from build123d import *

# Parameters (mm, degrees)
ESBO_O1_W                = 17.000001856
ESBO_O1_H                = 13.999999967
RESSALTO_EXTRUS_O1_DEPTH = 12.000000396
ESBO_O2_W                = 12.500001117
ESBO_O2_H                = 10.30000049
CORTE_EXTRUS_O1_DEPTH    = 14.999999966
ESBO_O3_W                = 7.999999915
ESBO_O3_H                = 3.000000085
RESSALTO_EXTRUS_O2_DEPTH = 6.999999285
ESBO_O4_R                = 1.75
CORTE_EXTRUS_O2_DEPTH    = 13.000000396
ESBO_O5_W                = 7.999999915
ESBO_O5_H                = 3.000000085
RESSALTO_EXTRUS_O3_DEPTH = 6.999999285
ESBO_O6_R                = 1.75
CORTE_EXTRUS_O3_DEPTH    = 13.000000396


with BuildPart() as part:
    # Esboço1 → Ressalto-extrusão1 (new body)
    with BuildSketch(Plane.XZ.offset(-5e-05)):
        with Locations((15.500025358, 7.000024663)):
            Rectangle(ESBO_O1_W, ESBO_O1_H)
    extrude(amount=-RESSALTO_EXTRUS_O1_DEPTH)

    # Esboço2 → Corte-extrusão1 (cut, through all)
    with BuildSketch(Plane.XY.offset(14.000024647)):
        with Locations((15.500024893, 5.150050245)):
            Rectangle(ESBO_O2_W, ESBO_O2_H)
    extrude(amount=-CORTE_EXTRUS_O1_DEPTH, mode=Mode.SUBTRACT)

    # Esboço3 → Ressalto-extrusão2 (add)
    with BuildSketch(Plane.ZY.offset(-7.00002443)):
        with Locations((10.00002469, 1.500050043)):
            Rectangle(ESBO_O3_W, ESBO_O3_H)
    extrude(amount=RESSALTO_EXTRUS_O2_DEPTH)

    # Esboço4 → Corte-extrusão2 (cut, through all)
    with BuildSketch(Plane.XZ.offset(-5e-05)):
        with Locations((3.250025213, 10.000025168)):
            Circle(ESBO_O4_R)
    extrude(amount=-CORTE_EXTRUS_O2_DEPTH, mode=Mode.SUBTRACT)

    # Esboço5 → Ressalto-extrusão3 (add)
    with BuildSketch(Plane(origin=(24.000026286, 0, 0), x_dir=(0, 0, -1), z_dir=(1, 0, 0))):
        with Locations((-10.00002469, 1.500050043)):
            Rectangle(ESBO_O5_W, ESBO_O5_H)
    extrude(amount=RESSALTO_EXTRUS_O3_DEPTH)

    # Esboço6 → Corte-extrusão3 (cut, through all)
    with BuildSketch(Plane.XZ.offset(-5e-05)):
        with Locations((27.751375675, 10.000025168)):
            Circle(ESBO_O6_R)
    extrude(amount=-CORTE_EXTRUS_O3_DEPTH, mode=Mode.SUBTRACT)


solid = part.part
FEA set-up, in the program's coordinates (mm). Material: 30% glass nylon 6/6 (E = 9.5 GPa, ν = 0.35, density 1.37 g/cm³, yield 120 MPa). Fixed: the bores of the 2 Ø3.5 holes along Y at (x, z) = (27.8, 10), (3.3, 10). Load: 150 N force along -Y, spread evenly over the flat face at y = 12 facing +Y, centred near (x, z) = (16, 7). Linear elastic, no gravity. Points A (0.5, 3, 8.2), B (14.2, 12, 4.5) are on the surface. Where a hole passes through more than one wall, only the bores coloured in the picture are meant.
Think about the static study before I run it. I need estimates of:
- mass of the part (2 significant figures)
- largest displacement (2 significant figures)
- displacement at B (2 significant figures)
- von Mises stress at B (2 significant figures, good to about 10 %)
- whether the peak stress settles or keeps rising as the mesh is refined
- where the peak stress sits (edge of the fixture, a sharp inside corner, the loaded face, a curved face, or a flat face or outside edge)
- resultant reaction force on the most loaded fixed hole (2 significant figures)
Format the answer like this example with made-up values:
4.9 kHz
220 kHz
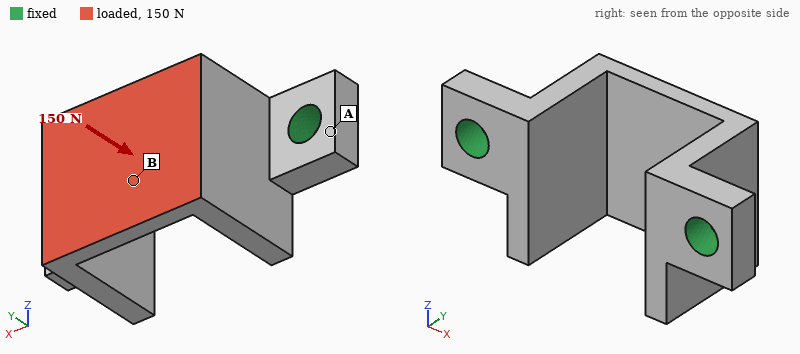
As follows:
1.8 g
80 µm
61 µm
11 MPa
keeps rising
edge of the fixture
80 N
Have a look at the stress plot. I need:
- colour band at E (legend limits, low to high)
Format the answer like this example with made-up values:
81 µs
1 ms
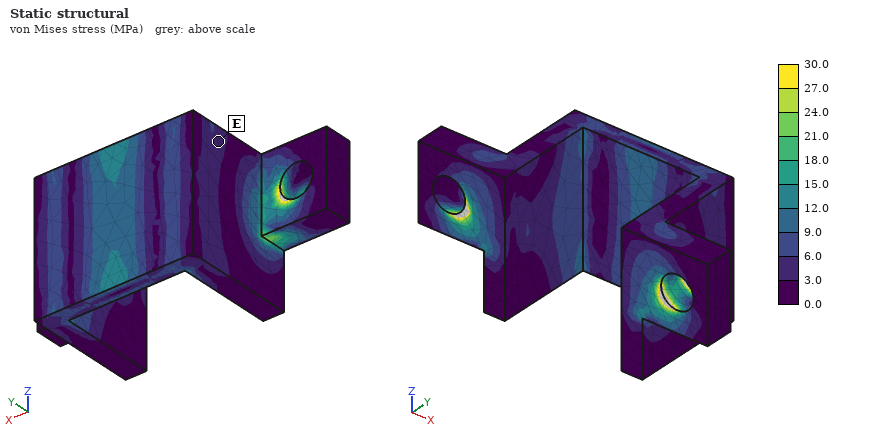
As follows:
3.0 to 6.0 MPa
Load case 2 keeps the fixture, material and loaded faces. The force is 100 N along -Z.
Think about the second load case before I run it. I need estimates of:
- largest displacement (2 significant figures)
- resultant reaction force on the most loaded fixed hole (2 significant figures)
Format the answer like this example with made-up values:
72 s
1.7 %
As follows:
0.13 mm
50 N
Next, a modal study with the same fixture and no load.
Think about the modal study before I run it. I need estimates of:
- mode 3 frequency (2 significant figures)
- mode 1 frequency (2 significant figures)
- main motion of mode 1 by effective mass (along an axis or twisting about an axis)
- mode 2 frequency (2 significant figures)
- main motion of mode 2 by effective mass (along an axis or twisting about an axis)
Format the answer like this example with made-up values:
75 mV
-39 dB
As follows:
7900 Hz
5300 Hz
along Z
6100 Hz
along X
